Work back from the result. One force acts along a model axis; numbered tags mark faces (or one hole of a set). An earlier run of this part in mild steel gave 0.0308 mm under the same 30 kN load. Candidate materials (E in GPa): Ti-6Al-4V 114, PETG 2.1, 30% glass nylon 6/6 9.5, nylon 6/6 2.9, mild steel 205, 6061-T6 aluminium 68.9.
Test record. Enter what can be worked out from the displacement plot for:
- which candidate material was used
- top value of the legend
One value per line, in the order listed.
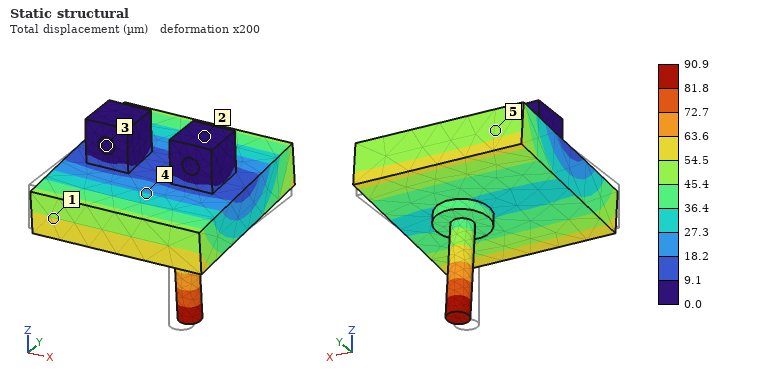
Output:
6061-T6 aluminium
90.9 µm
